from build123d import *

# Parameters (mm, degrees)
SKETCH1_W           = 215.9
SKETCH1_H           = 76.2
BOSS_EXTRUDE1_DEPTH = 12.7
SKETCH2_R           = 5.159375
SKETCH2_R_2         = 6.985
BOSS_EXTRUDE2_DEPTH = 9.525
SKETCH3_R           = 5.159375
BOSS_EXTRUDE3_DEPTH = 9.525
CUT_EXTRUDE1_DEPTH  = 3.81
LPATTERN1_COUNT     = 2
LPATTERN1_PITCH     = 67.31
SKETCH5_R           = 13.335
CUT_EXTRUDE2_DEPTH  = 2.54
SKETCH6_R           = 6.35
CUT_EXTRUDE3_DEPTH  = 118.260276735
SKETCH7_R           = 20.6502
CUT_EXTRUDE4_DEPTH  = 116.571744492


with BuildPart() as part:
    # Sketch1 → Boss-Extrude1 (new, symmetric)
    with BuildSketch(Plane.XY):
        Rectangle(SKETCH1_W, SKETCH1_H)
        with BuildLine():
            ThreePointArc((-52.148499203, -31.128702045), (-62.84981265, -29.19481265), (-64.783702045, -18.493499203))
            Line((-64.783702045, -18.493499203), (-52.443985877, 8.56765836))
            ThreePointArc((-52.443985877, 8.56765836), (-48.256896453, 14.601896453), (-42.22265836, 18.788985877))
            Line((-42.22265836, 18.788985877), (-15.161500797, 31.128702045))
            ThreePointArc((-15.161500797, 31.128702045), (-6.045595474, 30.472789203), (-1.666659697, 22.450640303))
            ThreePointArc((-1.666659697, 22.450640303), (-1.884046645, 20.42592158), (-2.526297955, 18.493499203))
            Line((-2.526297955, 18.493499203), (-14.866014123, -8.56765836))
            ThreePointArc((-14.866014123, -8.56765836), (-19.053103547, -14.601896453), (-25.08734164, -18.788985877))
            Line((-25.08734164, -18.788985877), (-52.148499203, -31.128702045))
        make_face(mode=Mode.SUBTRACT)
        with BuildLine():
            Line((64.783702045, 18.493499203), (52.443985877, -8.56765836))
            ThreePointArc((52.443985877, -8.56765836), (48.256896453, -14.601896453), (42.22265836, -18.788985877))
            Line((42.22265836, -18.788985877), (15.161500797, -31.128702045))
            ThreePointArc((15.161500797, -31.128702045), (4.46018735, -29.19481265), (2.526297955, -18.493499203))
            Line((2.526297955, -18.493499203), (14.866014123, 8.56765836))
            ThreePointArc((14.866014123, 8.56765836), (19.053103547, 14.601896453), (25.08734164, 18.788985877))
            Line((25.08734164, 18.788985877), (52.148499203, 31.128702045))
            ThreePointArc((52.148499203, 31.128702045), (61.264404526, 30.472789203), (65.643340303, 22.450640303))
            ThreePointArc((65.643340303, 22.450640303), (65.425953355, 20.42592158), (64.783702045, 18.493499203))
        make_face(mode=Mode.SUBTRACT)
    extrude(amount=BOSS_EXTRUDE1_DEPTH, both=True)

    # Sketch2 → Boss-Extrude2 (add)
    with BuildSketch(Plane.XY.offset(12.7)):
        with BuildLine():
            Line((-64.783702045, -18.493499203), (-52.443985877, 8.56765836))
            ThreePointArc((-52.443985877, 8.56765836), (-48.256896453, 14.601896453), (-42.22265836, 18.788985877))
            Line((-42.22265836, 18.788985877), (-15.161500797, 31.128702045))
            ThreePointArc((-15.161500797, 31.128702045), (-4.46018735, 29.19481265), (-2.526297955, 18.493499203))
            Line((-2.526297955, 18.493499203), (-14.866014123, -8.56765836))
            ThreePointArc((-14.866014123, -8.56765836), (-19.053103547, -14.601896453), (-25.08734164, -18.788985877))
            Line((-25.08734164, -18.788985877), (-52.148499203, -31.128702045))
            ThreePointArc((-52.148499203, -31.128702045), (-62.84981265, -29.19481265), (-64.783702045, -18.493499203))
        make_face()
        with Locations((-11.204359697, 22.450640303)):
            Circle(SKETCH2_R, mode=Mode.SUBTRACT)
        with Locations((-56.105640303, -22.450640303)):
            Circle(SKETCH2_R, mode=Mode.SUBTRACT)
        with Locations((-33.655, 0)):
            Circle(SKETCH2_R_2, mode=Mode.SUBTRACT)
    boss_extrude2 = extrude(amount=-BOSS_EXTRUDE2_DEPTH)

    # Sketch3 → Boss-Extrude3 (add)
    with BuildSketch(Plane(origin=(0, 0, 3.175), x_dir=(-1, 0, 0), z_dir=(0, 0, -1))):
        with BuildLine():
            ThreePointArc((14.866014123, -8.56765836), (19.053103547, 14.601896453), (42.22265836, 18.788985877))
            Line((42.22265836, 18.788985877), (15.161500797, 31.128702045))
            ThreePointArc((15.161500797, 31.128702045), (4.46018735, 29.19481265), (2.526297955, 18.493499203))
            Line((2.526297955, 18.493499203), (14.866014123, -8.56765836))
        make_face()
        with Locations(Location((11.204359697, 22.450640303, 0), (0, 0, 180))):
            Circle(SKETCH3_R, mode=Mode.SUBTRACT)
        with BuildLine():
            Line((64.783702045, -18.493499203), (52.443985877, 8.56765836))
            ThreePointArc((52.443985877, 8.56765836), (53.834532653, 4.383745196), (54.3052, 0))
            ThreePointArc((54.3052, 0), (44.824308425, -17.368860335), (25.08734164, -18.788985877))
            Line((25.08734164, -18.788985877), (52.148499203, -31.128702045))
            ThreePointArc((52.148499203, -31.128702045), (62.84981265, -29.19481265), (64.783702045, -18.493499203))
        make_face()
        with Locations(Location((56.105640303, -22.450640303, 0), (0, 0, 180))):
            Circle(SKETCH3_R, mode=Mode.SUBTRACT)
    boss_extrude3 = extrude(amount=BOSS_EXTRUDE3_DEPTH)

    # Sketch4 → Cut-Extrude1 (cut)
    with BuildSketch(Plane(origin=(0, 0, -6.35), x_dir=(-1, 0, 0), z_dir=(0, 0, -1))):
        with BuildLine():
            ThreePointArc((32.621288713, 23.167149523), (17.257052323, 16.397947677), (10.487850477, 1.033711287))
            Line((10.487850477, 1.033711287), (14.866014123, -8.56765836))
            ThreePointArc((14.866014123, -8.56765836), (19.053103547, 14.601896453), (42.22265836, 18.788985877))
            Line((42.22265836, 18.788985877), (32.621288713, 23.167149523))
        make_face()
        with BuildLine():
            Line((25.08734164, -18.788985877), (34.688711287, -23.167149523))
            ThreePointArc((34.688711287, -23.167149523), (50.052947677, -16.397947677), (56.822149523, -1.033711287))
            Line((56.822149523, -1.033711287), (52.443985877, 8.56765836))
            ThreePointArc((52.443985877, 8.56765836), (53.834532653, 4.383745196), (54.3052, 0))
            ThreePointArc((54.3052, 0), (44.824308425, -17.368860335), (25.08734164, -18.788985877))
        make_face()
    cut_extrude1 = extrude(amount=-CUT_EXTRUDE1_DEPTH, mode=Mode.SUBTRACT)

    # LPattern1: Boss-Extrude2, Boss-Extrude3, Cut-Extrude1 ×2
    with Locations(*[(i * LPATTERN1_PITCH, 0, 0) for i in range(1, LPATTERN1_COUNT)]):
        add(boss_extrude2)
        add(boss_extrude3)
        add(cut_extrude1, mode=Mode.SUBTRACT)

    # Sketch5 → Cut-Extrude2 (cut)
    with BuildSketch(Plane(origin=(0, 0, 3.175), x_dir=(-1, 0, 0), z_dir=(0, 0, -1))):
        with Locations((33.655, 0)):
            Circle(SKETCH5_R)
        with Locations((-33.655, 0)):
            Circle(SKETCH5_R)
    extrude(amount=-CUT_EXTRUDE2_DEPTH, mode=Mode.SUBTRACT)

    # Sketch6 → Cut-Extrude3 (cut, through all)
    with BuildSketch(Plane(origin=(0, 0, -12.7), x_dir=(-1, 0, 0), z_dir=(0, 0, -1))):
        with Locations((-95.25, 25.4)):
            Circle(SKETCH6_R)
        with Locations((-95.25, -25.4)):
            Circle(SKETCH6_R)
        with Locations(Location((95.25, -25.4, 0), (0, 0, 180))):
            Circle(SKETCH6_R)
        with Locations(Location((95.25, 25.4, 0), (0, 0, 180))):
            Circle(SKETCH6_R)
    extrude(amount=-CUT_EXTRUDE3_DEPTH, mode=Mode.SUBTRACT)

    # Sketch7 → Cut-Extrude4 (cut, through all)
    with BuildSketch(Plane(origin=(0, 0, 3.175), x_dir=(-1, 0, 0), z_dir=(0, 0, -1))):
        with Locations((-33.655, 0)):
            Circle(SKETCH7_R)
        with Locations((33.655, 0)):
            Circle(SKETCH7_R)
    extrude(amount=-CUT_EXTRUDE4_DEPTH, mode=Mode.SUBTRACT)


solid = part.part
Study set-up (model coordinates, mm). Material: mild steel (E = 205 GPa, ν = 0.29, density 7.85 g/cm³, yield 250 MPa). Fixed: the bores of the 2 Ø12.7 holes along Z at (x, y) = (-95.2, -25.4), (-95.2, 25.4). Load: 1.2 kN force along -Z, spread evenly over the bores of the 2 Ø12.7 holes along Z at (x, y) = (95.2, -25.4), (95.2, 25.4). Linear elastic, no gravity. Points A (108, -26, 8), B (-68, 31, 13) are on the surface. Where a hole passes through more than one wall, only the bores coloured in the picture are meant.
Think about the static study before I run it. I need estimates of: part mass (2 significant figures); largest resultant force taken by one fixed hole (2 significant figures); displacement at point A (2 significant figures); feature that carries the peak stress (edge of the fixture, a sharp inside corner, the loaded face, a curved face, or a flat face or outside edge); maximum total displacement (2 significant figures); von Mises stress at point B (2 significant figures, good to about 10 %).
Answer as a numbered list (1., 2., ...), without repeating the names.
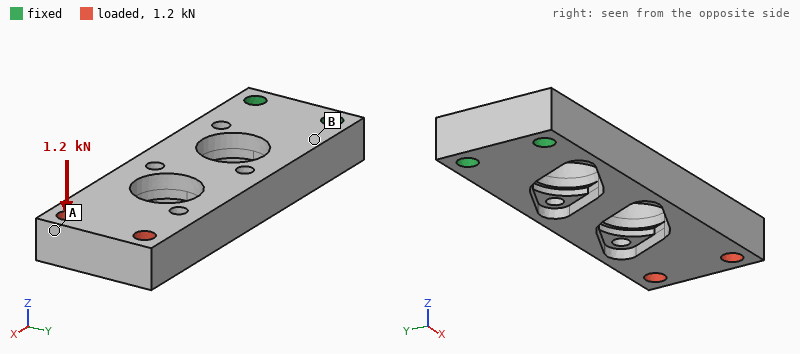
1. 2.5 kg
2. 660 N
3. 0.28 mm
4. a curved face
5. 0.29 mm
6. 30 MPa
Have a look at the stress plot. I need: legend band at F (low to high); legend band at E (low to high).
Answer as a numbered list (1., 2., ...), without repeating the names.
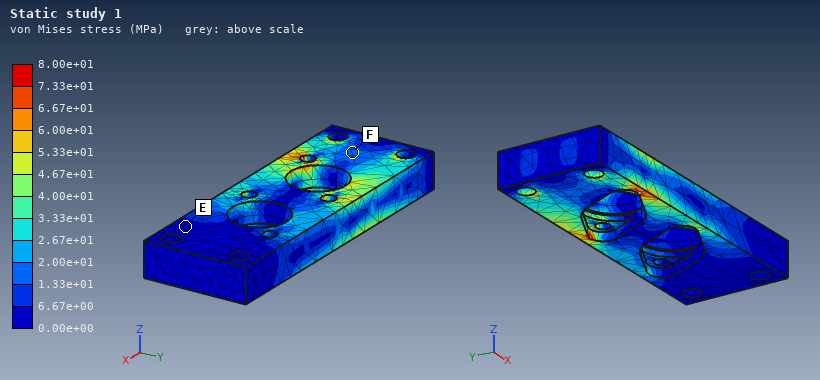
1. 1.33e+01 to 2.00e+01 MPa
2. 0.00e+00 to 6.67e+00 MPa
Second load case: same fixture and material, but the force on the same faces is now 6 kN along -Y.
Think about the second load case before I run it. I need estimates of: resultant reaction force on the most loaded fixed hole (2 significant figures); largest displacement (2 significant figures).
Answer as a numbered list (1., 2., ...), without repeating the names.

1. 20 kN
2. 0.14 mm
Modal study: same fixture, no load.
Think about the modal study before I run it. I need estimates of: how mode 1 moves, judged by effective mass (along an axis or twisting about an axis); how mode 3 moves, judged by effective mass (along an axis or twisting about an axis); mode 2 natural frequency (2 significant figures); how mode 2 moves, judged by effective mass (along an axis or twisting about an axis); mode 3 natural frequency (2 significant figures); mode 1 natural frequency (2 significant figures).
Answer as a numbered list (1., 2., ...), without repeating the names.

1. along Z
2. twisting about X
3. 1200 Hz
4. along Y
5. 1700 Hz
6. 410 Hz
